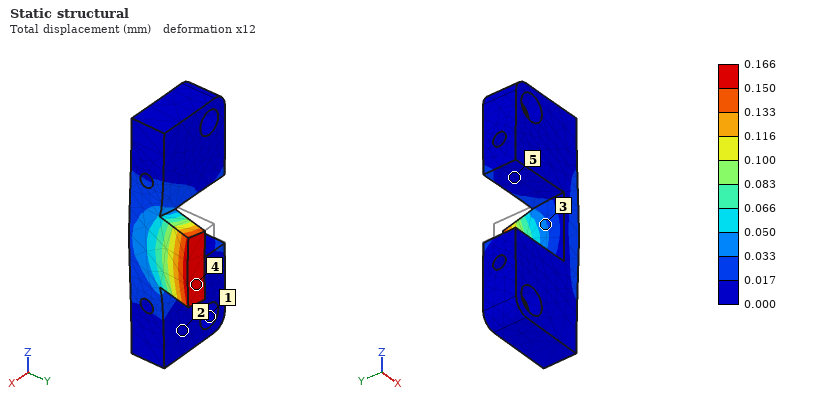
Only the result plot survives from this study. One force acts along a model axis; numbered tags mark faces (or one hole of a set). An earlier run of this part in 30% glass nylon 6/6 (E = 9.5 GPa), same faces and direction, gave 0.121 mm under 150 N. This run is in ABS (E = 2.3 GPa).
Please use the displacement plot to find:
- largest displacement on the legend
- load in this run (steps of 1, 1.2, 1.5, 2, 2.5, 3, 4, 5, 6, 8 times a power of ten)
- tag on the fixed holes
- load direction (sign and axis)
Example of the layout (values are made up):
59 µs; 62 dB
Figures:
0.166 mm; 50 N; 1; +X
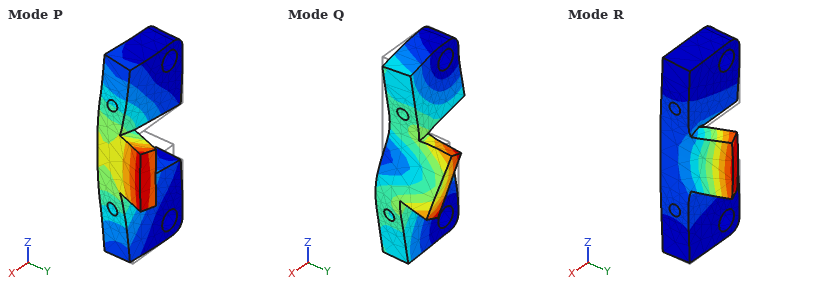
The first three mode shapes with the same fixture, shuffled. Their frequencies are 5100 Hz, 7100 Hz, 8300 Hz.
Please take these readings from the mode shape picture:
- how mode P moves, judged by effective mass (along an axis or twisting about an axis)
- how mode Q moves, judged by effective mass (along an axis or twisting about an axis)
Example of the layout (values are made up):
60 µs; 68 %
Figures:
along Y; along Z
